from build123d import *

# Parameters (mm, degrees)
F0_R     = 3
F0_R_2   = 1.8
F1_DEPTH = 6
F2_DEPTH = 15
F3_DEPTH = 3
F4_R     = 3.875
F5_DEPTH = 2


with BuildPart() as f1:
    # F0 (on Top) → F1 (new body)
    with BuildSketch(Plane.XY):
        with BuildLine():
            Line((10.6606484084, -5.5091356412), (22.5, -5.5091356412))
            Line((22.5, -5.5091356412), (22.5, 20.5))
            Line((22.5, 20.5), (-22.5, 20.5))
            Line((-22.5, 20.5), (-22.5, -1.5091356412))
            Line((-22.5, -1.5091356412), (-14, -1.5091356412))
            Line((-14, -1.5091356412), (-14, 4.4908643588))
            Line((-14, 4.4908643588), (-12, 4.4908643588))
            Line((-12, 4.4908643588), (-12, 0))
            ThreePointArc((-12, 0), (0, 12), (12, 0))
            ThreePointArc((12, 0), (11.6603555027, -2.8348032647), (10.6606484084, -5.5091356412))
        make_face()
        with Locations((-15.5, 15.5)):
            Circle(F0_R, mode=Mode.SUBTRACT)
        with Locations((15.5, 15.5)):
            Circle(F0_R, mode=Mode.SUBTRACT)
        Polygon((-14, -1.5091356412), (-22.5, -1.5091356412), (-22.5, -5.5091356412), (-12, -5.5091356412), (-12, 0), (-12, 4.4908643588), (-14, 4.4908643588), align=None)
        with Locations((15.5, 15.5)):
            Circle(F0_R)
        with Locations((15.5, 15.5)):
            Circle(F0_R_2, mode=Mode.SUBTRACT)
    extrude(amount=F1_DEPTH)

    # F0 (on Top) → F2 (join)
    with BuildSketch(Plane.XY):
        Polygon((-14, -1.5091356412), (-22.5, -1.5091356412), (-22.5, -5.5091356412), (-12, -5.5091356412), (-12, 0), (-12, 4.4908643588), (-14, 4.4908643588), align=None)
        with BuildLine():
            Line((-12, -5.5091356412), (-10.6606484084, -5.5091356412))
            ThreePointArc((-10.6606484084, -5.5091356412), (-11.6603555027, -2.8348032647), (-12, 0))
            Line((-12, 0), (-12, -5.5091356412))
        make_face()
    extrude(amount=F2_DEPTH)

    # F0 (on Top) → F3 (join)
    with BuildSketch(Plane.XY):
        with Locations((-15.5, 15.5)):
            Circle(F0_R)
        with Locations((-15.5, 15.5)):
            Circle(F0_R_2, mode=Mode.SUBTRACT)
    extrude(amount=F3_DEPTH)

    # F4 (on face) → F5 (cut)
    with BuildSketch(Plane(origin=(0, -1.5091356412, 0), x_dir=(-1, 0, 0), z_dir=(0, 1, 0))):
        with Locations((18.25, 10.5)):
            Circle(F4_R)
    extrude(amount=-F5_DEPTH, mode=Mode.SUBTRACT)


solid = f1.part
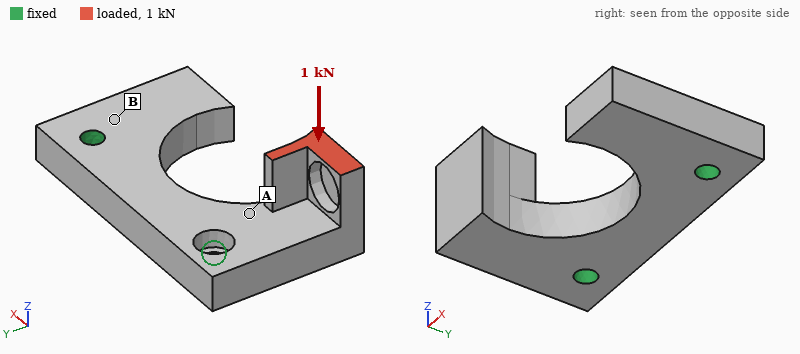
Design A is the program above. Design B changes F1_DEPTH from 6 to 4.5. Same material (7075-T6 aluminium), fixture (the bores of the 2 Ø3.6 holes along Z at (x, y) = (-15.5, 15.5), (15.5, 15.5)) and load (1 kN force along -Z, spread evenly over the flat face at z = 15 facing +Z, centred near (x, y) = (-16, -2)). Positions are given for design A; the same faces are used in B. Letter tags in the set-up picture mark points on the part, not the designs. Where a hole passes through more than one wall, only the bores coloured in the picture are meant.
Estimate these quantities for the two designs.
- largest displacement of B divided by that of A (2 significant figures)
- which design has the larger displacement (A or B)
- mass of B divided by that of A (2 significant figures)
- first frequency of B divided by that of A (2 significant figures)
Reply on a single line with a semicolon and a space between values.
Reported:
1.7; B; 0.79; 0.80
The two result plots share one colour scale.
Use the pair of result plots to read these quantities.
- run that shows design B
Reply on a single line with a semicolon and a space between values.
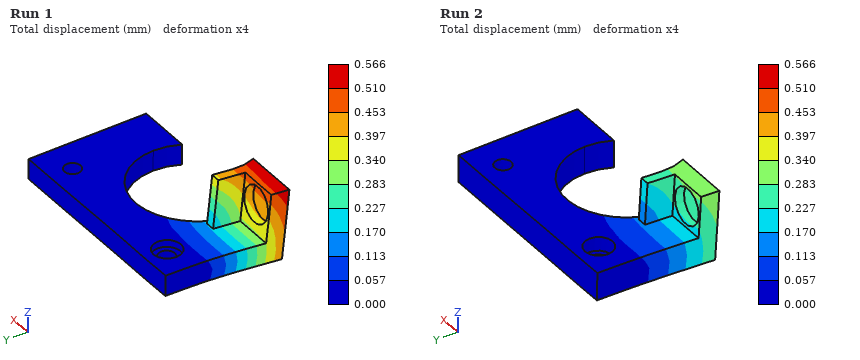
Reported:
Run 1
